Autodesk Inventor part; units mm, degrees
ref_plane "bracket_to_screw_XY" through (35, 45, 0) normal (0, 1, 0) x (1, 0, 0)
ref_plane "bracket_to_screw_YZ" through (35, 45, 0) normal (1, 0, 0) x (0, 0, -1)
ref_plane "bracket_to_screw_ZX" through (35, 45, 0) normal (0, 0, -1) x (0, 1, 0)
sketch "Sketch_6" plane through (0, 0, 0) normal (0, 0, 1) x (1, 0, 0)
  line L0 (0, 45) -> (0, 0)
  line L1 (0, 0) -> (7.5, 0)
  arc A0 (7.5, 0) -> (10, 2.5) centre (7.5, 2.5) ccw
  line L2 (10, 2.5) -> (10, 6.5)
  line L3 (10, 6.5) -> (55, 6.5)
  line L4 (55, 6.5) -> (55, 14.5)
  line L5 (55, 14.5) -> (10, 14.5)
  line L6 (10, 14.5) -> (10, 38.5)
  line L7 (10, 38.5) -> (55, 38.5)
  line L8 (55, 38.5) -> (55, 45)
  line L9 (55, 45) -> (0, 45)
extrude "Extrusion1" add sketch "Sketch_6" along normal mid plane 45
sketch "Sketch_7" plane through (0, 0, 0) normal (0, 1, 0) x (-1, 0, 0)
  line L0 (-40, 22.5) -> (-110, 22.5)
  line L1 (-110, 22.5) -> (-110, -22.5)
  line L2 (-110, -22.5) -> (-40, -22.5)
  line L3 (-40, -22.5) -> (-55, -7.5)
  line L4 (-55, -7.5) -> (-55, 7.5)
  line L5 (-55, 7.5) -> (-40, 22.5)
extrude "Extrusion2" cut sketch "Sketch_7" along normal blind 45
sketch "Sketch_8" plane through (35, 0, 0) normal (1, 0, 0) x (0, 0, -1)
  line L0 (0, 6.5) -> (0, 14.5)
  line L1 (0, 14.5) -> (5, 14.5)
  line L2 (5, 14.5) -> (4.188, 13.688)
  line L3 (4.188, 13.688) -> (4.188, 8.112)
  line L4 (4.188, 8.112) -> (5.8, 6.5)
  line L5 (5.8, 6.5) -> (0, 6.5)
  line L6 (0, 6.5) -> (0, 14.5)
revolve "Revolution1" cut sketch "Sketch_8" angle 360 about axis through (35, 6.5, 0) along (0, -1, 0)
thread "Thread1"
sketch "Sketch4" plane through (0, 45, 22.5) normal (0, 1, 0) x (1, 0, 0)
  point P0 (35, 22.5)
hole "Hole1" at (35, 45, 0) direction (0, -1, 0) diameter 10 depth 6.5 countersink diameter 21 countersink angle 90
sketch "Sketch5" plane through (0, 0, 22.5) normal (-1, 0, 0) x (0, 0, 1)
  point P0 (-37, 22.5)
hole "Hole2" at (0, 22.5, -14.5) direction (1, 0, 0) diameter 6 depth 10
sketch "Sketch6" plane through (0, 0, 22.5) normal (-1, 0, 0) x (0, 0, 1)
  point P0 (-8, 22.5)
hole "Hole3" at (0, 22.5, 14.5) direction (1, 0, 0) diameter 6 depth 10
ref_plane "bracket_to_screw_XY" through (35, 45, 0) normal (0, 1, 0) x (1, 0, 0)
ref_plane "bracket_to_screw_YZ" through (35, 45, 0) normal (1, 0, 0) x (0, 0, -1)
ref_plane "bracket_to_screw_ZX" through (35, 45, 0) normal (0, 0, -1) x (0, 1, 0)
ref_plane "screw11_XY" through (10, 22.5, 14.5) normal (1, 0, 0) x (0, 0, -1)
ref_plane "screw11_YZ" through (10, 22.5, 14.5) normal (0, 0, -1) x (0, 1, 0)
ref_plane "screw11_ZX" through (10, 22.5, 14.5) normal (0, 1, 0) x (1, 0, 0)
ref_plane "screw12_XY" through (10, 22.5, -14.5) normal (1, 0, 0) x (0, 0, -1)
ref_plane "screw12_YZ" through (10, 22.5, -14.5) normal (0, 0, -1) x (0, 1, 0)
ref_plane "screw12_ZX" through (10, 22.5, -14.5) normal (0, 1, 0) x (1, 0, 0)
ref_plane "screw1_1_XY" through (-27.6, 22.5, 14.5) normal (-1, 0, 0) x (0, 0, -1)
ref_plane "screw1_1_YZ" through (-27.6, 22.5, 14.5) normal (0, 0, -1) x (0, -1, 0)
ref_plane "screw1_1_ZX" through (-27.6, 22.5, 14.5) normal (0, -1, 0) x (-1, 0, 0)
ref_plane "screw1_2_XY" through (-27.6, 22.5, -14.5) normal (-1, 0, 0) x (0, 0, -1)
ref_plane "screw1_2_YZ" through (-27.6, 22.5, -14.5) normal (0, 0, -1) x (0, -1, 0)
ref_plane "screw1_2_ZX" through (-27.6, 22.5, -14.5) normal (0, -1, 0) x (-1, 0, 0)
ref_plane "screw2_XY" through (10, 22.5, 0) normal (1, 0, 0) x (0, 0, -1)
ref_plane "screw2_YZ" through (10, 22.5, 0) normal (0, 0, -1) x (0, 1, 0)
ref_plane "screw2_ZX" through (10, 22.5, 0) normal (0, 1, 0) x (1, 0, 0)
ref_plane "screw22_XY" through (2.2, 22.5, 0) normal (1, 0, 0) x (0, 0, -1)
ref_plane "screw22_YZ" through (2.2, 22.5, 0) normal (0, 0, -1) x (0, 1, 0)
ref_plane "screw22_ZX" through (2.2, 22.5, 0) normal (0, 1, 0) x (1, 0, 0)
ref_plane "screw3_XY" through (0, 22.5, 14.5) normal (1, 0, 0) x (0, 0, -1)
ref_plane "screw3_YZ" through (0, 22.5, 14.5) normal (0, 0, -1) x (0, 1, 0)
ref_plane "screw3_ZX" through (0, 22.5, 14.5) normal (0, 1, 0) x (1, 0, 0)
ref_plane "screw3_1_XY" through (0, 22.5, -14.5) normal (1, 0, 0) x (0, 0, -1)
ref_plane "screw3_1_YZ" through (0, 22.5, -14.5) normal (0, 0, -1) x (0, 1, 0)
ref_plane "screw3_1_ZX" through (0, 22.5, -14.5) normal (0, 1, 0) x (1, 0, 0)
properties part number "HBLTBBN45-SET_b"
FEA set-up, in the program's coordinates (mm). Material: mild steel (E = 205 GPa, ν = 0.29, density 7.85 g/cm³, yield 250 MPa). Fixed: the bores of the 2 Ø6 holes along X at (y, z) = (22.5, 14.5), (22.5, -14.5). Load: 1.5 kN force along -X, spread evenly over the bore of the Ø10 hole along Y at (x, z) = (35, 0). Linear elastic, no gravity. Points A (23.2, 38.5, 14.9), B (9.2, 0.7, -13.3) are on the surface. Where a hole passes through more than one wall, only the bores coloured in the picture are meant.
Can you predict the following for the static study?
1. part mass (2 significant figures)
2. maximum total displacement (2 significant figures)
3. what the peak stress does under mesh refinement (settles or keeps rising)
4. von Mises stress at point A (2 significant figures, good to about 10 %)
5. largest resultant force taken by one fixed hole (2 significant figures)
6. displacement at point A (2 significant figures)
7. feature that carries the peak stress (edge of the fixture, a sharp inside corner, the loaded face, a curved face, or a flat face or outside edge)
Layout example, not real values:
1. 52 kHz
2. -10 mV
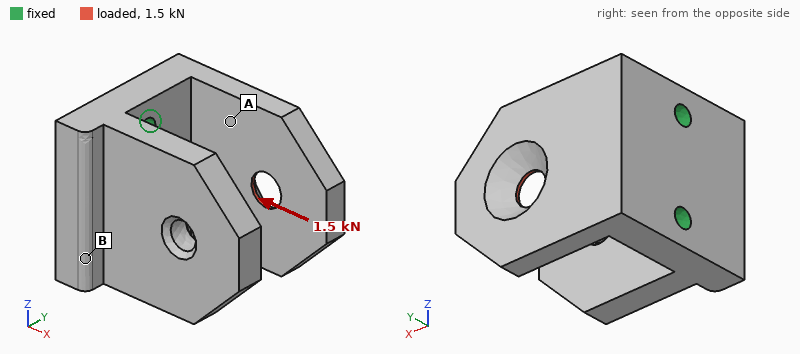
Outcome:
1. 350 g
2. 7.9 µm
3. keeps rising
4. 17 MPa
5. 750 N
6. 5.7 µm
7. a sharp inside corner
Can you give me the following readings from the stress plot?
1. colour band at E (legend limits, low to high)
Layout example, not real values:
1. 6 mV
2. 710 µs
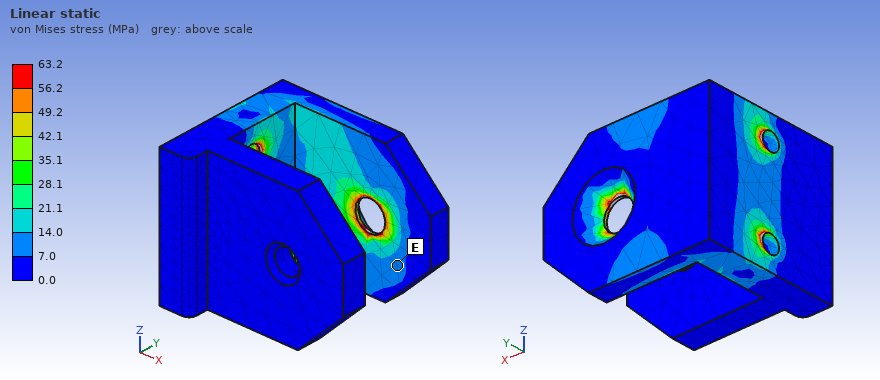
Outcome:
1. 7.0 to 14.0 MPa
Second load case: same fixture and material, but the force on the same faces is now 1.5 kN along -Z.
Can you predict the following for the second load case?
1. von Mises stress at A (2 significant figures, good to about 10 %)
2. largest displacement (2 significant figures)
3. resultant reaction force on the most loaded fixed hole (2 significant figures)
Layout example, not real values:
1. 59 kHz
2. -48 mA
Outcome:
1. 22 MPa
2. 27 µm
3. 1.7 kN
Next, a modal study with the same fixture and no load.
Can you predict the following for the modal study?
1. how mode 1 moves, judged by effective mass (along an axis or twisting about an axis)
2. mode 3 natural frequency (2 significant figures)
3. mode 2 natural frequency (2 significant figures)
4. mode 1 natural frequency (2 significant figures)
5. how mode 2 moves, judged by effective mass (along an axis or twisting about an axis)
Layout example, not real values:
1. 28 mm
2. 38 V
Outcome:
1. along Y
2. 5300 Hz
3. 2800 Hz
4. 2400 Hz
5. along Y
